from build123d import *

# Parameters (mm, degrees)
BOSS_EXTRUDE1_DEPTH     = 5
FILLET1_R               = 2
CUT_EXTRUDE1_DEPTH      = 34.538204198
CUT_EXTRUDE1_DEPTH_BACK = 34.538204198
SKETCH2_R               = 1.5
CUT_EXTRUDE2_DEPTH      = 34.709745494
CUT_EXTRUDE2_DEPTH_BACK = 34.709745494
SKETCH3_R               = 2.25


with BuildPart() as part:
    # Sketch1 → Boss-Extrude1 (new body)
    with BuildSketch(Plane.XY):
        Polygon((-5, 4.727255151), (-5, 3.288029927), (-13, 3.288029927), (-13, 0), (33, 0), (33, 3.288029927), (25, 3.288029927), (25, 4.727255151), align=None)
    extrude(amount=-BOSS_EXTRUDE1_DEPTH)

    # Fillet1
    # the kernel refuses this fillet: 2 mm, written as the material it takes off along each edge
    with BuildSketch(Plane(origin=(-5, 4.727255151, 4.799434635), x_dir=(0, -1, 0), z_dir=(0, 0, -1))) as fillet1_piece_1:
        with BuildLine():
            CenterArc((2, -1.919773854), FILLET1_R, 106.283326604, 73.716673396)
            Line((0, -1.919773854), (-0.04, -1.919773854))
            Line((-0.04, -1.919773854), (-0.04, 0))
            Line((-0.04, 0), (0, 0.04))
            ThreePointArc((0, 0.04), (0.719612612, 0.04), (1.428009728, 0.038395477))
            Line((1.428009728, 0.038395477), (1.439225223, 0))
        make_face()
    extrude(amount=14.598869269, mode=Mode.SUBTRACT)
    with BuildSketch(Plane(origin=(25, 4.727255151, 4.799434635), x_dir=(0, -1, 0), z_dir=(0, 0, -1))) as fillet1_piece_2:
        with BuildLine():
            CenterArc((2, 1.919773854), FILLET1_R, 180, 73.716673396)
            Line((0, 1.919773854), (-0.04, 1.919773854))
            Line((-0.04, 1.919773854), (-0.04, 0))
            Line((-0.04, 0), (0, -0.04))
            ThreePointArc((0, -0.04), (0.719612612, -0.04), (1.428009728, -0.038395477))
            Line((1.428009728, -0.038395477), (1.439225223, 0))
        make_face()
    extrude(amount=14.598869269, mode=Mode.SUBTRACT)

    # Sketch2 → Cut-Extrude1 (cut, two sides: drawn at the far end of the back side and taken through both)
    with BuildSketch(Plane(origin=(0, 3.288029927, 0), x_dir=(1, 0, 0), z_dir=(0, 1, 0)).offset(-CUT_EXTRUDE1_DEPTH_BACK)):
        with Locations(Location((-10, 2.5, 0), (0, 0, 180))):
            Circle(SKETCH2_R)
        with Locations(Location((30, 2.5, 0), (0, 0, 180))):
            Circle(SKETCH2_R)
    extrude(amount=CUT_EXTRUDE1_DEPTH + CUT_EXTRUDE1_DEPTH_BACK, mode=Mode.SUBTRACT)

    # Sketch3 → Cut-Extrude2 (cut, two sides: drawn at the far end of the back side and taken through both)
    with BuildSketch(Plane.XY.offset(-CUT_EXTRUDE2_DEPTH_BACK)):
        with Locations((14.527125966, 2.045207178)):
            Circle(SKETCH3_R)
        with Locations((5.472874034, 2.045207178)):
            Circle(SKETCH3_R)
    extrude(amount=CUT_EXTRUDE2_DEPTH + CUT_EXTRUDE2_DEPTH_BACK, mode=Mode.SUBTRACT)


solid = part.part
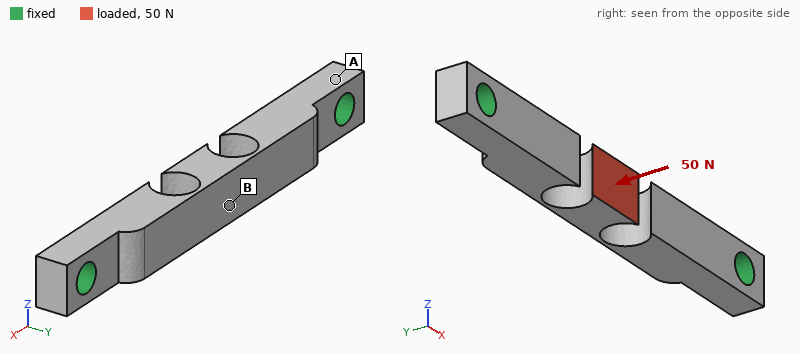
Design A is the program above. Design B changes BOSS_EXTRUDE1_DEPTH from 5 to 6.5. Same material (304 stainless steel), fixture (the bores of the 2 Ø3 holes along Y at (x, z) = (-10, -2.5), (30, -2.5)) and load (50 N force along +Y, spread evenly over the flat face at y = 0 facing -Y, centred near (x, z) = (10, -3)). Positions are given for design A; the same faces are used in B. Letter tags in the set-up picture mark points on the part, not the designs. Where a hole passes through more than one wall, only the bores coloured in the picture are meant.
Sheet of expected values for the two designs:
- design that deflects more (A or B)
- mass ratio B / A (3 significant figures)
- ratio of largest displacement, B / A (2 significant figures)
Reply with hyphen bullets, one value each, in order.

- A
- 1.32
- 0.79
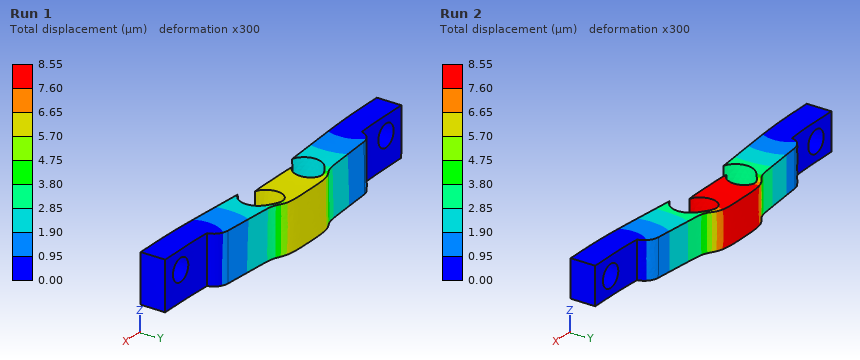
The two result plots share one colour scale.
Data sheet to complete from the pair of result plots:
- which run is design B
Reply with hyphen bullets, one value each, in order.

- Run 1
